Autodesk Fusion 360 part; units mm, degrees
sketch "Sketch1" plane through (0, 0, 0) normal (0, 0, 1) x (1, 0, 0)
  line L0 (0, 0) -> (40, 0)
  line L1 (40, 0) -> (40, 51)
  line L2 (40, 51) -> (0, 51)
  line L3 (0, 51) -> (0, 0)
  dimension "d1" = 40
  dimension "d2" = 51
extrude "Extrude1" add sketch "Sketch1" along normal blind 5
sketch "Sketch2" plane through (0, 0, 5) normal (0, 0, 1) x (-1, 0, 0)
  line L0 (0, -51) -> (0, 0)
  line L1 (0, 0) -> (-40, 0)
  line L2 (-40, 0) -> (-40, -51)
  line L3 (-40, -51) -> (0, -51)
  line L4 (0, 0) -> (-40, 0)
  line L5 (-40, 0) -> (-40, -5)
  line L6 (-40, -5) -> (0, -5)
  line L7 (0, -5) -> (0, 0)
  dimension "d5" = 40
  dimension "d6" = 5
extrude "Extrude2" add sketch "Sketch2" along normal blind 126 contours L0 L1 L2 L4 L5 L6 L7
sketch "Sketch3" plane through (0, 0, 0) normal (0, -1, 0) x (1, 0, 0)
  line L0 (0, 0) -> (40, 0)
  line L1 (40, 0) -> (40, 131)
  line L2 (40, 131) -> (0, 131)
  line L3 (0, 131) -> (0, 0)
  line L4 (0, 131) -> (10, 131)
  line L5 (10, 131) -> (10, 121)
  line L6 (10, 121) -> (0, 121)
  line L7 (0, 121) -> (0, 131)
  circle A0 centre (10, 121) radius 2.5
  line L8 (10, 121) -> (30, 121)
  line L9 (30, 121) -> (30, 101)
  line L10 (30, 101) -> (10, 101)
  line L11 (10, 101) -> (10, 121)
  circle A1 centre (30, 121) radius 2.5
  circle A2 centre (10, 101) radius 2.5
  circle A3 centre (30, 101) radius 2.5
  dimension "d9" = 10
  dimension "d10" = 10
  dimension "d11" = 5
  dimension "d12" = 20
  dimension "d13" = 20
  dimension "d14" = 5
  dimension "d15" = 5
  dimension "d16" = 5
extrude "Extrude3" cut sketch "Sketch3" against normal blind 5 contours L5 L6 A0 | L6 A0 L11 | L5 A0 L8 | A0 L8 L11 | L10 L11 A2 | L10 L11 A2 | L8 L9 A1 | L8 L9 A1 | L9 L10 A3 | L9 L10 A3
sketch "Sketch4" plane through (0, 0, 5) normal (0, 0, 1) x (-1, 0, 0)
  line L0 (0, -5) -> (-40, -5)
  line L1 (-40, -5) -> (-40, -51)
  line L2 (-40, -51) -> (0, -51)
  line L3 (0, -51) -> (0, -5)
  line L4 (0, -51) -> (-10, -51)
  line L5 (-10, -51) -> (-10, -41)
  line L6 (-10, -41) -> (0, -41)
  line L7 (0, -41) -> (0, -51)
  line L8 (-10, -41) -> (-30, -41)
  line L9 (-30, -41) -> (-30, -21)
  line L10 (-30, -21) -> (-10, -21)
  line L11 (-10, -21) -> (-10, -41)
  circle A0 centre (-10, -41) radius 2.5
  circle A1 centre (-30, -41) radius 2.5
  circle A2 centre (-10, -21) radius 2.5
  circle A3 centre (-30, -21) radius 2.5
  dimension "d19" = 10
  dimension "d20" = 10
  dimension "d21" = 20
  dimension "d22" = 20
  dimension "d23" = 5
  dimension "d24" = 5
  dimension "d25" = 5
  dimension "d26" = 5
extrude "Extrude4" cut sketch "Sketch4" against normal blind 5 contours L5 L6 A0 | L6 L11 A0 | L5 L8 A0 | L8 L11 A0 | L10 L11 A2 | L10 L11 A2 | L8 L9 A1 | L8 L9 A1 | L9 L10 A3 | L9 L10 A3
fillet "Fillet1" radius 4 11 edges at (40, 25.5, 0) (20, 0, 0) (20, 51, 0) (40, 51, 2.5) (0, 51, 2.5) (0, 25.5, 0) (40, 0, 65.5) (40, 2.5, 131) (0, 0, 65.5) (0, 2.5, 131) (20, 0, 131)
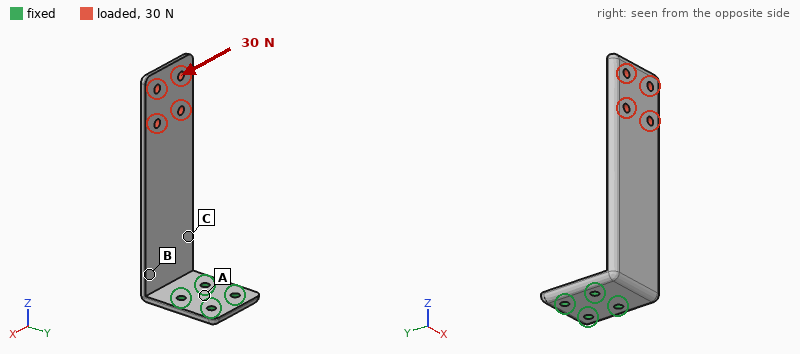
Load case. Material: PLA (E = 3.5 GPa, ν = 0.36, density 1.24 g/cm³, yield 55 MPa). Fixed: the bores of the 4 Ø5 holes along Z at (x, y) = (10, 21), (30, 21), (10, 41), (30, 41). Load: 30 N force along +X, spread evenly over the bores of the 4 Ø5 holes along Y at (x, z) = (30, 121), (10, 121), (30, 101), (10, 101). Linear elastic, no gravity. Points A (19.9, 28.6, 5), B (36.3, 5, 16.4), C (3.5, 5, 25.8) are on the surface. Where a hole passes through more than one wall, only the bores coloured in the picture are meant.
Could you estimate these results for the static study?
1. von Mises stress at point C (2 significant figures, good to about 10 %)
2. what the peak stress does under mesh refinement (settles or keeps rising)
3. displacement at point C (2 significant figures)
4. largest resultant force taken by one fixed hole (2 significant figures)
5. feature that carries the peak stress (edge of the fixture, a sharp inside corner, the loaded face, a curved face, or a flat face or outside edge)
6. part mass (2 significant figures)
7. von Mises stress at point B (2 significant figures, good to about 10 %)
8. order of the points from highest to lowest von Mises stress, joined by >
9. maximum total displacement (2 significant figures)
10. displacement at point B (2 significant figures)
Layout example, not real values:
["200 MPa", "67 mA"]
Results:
["2.7 MPa", "keeps rising", "0.38 mm", "140 N", "edge of the fixture", "41 g", "4.4 MPa", "B > C > A", "1.8 mm", "0.28 mm"]
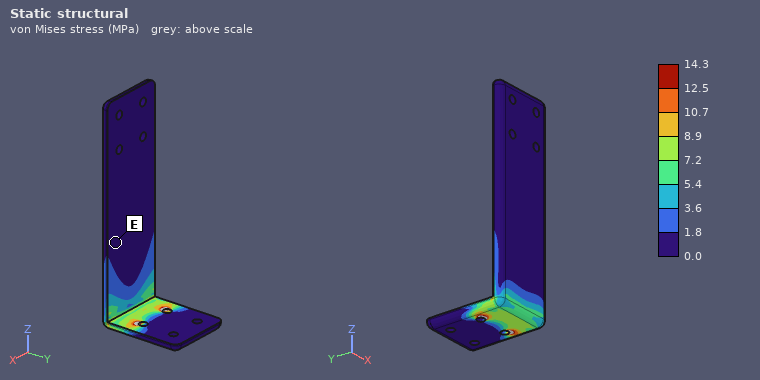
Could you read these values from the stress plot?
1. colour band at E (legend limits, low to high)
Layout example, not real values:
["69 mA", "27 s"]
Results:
["0.0 to 1.8 MPa"]
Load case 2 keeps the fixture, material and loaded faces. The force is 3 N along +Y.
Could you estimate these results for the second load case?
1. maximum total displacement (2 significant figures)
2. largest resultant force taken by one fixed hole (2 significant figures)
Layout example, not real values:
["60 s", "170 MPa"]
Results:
["1.6 mm", "3.8 N"]
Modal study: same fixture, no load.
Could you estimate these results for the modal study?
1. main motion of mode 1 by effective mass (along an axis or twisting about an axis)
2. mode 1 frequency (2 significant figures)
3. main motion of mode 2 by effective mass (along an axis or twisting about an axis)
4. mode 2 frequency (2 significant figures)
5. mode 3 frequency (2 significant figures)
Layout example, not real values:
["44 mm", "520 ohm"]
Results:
["along Y", "70 Hz", "along X", "200 Hz", "440 Hz"]
